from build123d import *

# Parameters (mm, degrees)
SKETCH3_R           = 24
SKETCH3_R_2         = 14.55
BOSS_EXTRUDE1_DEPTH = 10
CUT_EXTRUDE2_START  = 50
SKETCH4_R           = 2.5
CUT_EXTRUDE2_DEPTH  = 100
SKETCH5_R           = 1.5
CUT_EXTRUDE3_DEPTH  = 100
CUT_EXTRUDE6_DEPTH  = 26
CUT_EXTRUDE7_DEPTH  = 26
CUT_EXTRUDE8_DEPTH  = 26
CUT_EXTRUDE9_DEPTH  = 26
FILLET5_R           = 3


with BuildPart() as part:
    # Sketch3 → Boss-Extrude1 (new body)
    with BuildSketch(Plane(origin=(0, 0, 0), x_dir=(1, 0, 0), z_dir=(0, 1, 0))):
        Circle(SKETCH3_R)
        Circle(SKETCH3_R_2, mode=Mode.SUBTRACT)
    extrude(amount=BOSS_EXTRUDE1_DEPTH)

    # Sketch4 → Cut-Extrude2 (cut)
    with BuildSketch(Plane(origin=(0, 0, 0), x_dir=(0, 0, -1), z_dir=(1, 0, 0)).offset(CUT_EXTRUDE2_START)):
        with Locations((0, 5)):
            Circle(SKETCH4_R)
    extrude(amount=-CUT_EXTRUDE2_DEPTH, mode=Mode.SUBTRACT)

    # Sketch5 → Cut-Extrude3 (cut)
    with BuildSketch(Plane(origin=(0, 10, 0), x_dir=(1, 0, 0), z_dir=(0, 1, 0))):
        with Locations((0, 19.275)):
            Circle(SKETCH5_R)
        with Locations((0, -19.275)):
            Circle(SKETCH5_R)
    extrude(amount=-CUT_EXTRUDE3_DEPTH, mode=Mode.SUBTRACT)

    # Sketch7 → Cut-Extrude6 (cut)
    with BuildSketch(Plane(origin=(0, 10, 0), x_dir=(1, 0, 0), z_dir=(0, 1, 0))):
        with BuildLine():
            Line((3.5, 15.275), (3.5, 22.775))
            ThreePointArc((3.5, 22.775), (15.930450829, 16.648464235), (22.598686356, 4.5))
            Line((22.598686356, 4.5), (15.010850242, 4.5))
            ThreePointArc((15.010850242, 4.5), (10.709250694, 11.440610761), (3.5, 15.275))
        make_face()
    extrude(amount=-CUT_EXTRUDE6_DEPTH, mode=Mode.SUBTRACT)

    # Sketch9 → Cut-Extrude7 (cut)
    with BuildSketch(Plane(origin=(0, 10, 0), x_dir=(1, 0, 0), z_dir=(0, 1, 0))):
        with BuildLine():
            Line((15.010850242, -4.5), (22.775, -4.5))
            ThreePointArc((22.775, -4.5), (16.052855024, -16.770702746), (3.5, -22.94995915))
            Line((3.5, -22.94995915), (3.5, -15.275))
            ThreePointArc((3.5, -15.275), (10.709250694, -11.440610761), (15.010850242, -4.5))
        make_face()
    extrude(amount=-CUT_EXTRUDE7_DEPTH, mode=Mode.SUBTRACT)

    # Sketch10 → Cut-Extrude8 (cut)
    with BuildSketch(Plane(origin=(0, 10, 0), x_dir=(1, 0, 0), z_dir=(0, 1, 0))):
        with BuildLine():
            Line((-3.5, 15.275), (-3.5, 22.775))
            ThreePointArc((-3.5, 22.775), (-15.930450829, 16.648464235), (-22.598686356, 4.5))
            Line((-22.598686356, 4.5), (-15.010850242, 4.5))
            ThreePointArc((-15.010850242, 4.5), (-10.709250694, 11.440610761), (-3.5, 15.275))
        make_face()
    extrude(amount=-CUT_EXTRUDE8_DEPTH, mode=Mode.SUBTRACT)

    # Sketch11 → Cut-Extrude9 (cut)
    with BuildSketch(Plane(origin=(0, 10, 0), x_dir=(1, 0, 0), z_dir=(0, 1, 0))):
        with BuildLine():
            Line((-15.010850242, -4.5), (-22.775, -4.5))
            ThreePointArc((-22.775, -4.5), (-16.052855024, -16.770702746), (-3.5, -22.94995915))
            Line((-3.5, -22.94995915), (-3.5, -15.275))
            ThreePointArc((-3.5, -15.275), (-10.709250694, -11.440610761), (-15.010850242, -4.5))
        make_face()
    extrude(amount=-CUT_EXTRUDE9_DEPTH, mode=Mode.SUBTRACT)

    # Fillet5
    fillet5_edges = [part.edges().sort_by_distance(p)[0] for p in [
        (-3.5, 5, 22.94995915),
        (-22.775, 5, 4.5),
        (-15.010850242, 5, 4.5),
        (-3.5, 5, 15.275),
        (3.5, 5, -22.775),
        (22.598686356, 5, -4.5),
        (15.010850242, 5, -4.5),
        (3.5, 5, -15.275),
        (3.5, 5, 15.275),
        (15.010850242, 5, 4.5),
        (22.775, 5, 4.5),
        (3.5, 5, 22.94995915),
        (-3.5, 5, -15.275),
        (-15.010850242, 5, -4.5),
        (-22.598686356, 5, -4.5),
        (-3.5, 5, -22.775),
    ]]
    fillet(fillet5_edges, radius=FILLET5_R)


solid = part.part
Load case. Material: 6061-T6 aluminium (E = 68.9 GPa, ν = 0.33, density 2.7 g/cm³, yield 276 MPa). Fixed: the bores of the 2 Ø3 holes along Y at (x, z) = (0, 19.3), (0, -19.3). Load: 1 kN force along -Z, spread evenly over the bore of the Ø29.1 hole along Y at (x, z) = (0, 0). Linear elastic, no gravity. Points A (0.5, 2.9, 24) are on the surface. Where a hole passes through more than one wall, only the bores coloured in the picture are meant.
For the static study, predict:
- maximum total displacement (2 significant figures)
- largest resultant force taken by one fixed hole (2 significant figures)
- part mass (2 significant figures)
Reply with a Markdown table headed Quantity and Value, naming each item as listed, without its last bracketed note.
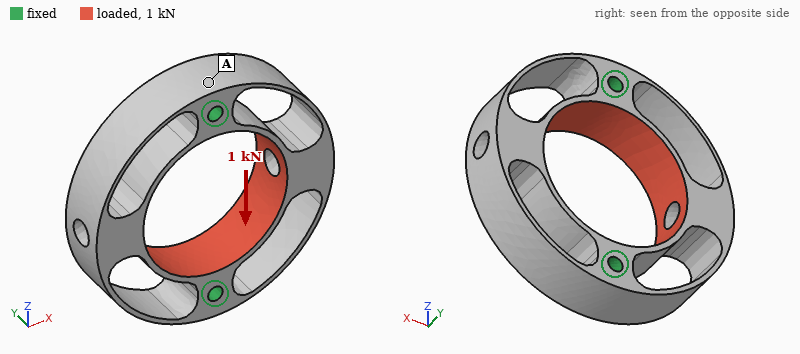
| Quantity | Value |
|---|---|
| maximum total displacement | 94 µm |
| largest resultant force taken by one fixed hole | 500 N |
| part mass | 12 g |
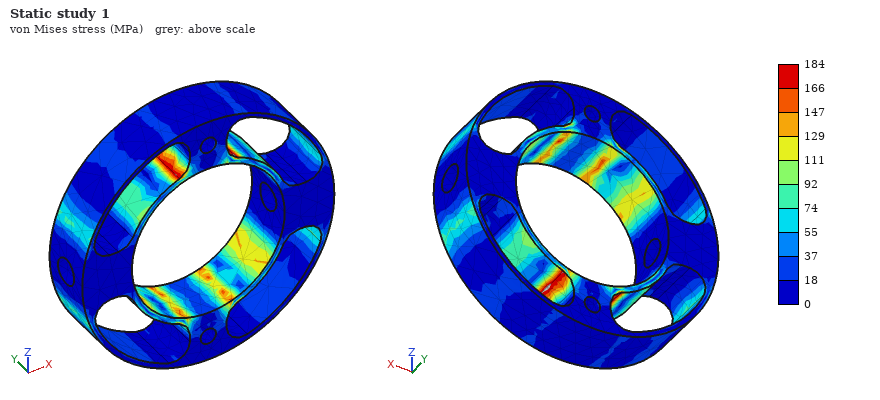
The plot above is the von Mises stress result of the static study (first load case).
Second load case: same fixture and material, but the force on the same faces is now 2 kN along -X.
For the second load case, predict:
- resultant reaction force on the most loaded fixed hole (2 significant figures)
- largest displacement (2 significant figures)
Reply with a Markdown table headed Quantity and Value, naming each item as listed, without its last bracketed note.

| Quantity | Value |
|---|---|
| resultant reaction force on the most loaded fixed hole | 1.0 kN |
| largest displacement | 16 µm |
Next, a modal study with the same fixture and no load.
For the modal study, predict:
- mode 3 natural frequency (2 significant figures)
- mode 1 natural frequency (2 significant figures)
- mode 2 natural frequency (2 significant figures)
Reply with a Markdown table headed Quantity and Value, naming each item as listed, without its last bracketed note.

| Quantity | Value |
|---|---|
| mode 3 natural frequency | 7600 Hz |
| mode 1 natural frequency | 5200 Hz |
| mode 2 natural frequency | 5300 Hz |
